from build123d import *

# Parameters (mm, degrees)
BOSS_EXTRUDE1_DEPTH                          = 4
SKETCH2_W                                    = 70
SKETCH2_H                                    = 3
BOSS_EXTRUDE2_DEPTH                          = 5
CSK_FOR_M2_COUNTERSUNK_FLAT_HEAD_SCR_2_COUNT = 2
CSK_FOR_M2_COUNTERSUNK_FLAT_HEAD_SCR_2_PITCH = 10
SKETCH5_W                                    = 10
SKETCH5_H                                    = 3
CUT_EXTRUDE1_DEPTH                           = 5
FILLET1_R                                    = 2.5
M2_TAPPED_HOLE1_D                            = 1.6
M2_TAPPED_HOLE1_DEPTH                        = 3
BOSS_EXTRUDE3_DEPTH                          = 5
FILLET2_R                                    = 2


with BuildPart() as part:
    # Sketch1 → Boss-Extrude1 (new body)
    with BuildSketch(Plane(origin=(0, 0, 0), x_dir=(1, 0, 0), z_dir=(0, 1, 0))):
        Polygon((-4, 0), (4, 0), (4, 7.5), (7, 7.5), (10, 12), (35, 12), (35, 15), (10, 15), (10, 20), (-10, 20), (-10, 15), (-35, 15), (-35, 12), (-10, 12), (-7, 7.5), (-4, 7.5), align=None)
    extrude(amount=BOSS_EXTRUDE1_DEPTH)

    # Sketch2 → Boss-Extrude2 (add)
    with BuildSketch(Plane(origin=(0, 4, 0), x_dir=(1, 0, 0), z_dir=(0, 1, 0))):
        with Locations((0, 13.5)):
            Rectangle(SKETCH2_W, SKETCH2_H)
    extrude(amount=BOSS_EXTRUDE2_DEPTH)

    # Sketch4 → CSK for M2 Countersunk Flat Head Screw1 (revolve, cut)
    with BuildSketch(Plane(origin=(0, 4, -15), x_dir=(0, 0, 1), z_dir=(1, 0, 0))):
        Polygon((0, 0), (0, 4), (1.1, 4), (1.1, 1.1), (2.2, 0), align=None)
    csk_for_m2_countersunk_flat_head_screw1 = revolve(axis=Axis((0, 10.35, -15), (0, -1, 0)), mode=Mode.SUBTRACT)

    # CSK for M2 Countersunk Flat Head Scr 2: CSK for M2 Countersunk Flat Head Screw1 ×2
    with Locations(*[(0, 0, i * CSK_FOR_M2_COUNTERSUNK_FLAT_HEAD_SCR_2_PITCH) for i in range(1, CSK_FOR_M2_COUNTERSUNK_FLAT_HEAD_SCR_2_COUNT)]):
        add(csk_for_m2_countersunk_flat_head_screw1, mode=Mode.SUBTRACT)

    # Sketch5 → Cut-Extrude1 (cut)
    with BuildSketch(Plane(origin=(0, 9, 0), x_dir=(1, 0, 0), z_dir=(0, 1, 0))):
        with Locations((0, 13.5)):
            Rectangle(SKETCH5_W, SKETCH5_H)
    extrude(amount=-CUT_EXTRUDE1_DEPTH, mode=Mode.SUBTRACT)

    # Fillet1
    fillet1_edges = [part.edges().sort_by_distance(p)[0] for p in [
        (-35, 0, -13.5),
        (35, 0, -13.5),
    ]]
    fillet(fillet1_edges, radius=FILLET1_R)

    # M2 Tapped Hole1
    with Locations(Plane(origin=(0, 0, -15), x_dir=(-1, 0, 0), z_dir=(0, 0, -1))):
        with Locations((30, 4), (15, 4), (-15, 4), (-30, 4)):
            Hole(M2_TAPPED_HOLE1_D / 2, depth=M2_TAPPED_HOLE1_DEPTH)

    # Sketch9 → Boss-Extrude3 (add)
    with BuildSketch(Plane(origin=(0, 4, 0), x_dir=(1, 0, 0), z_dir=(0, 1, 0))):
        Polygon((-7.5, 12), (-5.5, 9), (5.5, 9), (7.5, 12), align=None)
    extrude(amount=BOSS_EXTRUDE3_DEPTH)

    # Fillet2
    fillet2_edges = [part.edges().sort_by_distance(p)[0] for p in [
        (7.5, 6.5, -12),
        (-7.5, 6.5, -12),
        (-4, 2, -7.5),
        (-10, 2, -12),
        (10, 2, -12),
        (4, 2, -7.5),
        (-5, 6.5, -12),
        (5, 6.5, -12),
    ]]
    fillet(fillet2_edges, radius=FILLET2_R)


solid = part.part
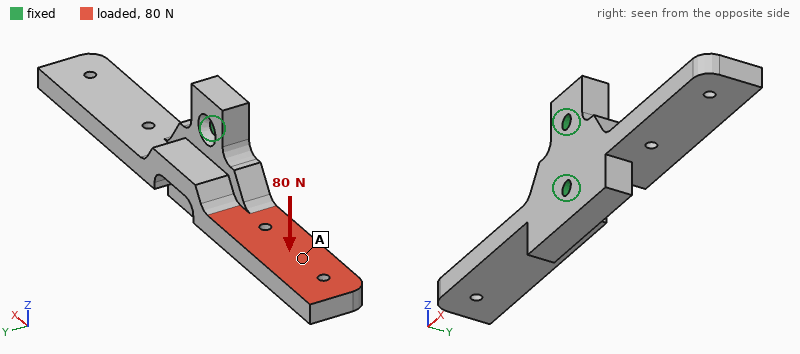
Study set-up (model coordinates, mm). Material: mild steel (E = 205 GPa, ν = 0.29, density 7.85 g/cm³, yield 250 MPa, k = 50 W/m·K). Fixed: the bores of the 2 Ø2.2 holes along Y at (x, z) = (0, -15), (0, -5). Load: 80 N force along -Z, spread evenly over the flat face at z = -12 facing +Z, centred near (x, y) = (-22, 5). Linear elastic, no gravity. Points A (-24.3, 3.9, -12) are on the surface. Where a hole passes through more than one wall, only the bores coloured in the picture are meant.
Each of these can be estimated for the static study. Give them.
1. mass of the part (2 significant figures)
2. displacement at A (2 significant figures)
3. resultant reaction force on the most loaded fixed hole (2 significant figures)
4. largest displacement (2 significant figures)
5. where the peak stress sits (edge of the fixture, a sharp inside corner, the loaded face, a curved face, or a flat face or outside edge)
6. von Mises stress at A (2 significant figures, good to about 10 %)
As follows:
22 g
26 µm
170 N
54 µm
the loaded face
14 MPa
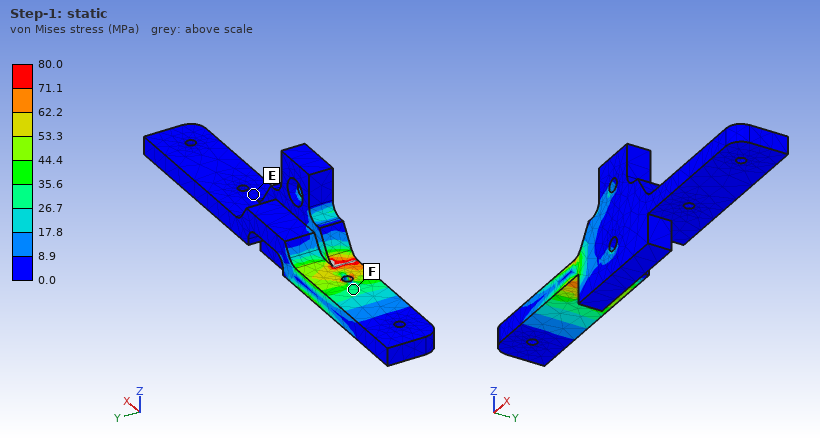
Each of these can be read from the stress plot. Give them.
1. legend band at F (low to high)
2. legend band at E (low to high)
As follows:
26.7 to 35.6 MPa
0.0 to 8.9 MPa
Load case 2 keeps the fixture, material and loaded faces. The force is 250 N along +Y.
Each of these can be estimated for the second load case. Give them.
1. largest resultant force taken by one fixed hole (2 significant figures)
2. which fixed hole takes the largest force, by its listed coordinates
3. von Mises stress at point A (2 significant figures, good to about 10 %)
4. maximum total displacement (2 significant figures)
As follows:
220 N
(0, -15)
23 MPa
85 µm
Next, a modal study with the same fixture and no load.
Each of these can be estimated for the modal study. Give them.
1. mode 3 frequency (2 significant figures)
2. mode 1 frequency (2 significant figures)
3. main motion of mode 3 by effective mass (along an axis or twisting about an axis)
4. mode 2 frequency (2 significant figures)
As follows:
3900 Hz
3300 Hz
twisting about Z
3400 Hz
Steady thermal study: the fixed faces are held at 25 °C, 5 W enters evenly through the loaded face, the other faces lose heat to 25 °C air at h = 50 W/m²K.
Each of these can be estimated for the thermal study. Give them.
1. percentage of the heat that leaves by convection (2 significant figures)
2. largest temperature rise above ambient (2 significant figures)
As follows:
24 %
55 K
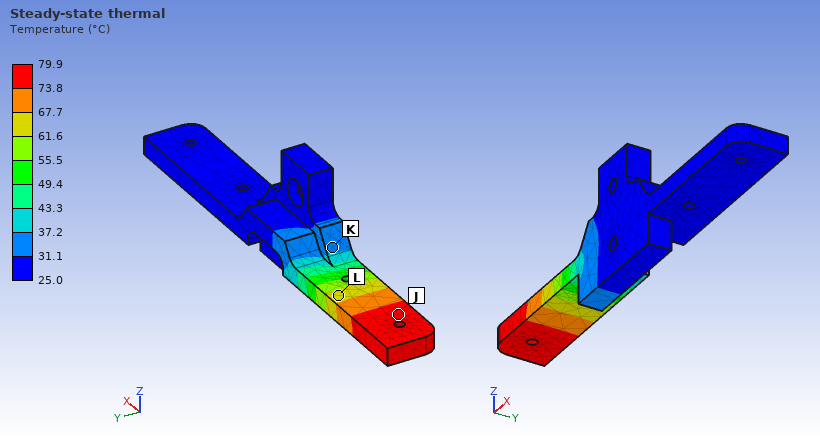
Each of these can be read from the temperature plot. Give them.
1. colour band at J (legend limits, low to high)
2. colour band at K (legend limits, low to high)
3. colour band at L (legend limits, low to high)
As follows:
73.8 to 79.9 °C
31.1 to 37.2 °C
61.6 to 67.7 °C
